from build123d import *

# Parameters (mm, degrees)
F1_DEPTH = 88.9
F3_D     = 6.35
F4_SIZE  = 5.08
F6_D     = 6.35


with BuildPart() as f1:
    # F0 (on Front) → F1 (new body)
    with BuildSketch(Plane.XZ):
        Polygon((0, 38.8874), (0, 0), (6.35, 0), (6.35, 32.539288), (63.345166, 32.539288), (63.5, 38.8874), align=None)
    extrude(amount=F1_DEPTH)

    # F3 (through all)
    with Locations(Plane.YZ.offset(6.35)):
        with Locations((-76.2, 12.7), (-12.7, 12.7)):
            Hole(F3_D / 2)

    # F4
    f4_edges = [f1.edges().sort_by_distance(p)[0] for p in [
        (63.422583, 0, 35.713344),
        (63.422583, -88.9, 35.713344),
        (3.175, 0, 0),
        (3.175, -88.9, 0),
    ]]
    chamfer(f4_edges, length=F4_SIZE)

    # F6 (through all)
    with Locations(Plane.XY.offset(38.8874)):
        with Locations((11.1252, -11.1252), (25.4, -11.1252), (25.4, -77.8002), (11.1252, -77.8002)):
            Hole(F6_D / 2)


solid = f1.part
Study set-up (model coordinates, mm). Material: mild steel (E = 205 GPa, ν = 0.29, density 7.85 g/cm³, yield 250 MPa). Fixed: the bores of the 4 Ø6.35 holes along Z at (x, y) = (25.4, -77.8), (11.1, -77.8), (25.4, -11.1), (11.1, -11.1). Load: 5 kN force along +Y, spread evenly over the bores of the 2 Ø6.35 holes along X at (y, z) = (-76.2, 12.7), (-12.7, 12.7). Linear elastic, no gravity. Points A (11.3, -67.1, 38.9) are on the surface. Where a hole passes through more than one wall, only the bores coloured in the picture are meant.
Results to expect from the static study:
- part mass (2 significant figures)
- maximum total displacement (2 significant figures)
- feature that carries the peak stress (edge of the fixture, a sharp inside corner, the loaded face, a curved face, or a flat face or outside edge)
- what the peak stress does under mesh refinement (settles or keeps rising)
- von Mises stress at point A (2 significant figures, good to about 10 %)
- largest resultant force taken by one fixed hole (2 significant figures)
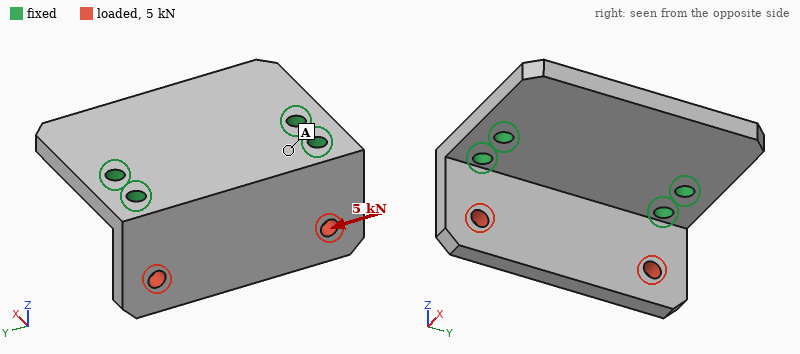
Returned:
410 g
12 µm
edge of the fixture
keeps rising
11 MPa
2.7 kN
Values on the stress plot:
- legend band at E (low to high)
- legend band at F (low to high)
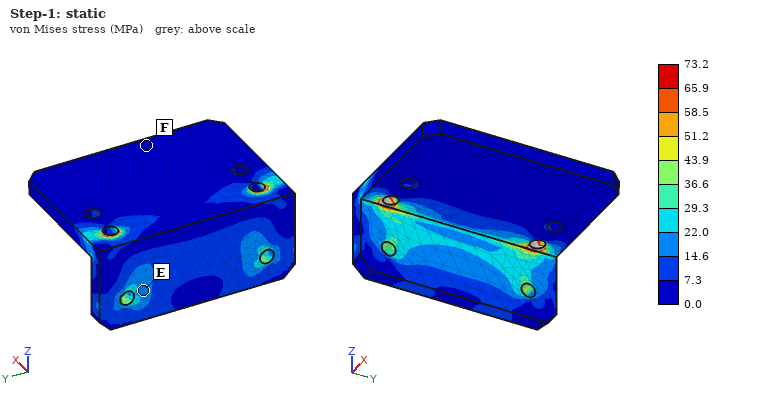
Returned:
14.6 to 22.0 MPa
0.0 to 7.3 MPa
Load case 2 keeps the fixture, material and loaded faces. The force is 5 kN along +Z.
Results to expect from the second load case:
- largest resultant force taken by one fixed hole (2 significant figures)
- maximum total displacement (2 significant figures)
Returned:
2.8 kN
21 µm
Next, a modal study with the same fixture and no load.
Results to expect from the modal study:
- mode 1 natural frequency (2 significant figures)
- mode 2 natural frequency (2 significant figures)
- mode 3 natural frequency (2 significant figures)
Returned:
3000 Hz
3200 Hz
4900 Hz
